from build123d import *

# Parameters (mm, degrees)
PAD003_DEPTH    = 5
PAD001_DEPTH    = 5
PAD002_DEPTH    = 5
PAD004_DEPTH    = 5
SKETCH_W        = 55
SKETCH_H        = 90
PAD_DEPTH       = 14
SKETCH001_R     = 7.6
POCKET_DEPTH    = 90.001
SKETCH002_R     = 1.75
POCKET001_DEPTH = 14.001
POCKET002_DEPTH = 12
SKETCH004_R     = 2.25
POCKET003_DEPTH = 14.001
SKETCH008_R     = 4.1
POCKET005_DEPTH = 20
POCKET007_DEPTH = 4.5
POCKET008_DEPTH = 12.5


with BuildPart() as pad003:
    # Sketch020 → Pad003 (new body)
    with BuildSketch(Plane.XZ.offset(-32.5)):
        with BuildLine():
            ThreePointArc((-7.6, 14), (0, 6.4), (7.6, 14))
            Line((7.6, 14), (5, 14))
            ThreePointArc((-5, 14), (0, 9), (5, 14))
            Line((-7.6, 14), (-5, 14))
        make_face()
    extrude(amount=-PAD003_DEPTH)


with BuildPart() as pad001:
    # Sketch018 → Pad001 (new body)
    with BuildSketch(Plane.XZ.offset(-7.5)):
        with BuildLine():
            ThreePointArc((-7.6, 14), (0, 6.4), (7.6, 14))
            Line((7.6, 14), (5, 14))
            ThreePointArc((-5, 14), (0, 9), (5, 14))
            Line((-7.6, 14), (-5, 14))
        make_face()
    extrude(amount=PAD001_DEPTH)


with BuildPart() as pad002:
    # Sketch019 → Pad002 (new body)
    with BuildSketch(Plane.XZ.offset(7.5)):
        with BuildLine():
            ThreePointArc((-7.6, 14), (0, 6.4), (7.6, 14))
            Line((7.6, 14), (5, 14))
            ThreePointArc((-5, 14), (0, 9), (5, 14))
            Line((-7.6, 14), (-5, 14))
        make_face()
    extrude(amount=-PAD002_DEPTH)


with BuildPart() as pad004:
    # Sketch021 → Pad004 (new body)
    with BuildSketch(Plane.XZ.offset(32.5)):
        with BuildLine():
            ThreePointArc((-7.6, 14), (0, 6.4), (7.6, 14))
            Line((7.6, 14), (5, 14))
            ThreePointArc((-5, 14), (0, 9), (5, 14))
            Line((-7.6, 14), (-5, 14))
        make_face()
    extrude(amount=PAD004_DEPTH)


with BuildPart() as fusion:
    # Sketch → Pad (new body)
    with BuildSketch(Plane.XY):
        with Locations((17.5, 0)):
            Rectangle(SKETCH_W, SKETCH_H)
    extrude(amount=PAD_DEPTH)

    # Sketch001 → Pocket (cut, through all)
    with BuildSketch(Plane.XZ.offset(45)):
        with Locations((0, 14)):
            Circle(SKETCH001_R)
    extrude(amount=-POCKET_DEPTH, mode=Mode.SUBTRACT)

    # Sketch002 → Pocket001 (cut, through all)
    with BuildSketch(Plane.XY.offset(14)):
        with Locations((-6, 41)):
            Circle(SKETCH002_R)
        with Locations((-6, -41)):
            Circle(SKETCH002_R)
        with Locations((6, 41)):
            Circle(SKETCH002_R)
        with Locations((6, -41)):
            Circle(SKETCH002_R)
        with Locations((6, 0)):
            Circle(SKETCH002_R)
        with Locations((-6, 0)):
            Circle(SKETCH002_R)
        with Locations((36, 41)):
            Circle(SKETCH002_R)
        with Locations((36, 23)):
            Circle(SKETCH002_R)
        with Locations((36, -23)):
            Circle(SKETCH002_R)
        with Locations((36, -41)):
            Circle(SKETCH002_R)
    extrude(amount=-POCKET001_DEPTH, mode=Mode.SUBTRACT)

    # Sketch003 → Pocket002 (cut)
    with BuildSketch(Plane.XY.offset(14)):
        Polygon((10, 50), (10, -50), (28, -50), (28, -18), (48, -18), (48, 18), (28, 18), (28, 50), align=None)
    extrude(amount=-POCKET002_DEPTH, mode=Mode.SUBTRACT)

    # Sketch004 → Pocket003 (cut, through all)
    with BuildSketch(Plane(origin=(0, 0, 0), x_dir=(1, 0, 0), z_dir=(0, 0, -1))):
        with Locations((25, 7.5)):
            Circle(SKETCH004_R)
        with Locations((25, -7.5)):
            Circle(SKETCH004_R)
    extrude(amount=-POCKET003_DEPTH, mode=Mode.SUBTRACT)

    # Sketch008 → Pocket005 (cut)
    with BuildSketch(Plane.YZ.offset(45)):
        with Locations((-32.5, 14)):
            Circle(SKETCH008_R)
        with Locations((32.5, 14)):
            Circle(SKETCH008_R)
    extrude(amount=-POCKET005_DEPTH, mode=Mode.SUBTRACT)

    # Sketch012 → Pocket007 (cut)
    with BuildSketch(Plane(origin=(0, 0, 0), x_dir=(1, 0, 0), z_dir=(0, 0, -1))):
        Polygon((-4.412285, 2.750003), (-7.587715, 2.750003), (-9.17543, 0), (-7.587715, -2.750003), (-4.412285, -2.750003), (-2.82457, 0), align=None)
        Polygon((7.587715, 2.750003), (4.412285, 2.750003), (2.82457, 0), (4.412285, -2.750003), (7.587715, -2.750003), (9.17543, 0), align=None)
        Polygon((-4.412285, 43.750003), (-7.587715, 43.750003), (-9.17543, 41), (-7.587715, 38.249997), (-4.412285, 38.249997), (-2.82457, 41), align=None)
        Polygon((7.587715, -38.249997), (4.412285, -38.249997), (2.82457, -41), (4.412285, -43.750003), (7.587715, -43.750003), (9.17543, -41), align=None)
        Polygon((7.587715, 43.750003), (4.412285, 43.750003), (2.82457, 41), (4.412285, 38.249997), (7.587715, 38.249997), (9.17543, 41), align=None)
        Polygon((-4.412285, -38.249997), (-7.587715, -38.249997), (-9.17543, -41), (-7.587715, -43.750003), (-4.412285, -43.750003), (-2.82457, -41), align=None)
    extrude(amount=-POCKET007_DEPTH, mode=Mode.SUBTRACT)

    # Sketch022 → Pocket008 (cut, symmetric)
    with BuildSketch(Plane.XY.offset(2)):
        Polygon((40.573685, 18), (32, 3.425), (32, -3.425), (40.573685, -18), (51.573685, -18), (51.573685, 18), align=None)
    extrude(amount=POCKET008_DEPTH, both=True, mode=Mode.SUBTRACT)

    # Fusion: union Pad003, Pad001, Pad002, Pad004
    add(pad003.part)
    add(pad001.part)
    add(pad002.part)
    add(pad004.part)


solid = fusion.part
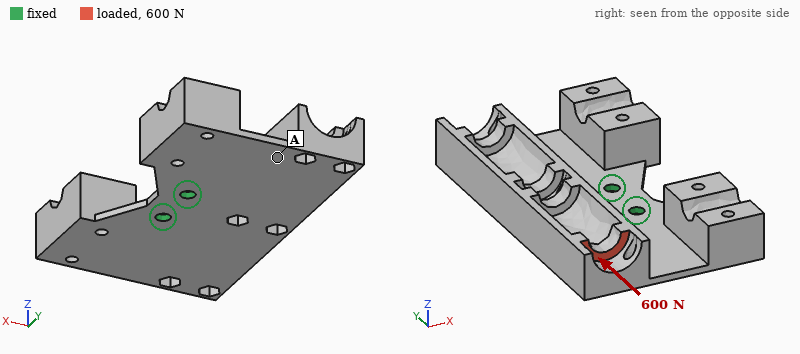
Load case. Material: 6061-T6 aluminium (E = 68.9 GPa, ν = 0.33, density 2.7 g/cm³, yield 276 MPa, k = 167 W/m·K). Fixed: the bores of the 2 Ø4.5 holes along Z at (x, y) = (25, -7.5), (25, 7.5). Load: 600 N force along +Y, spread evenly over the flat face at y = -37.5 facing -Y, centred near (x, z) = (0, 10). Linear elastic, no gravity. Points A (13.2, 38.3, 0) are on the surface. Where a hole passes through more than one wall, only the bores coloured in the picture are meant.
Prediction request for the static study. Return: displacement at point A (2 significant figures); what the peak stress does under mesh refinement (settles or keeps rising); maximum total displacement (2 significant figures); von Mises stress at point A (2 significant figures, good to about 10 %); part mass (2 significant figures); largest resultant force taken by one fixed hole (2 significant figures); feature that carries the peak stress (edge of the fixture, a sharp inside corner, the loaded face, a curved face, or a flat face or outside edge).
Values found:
0.20 mm
keeps rising
0.28 mm
15 MPa
87 g
860 N
edge of the fixture
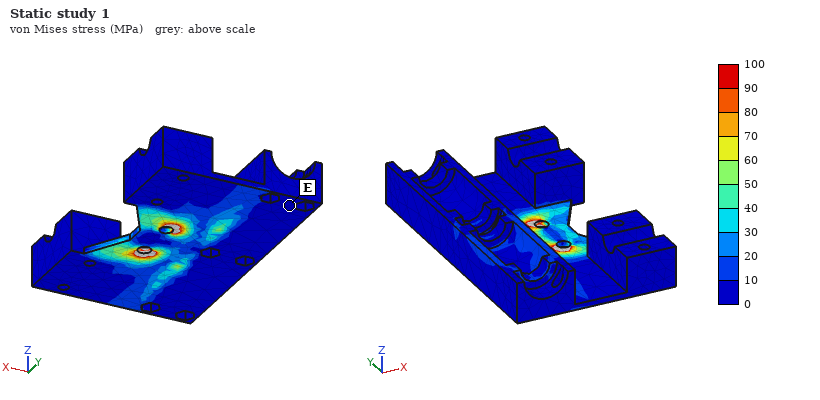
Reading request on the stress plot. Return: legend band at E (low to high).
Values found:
0 to 10 MPa
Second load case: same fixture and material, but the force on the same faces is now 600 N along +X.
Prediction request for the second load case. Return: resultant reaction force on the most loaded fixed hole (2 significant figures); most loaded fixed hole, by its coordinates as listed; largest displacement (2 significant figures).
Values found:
1.5 kN
(25, -7.5)
0.83 mm
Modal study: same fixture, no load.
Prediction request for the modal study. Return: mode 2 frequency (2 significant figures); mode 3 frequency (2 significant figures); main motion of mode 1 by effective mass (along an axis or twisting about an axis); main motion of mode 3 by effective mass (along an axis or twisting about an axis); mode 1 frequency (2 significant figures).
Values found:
630 Hz
910 Hz
along Z
along Z
510 Hz
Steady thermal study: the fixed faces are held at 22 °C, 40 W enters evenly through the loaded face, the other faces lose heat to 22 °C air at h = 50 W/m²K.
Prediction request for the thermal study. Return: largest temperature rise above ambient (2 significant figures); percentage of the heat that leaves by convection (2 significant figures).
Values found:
62 K
42 %
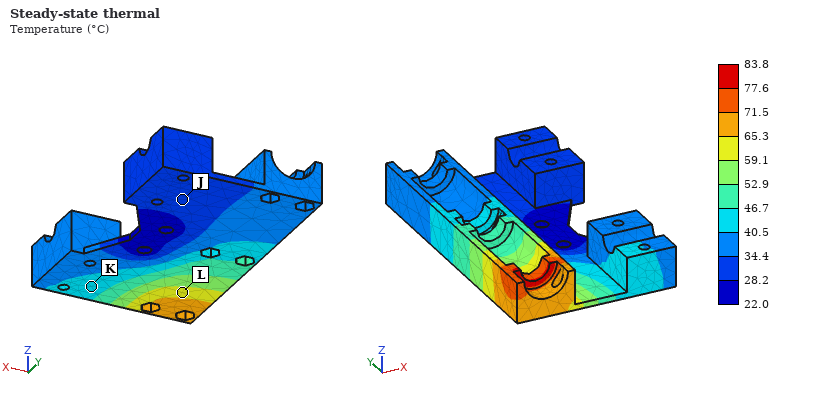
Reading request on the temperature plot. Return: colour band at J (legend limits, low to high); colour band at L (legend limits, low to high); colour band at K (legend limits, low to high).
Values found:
28.2 to 34.4 °C
59.1 to 65.3 °C
40.5 to 46.7 °C
